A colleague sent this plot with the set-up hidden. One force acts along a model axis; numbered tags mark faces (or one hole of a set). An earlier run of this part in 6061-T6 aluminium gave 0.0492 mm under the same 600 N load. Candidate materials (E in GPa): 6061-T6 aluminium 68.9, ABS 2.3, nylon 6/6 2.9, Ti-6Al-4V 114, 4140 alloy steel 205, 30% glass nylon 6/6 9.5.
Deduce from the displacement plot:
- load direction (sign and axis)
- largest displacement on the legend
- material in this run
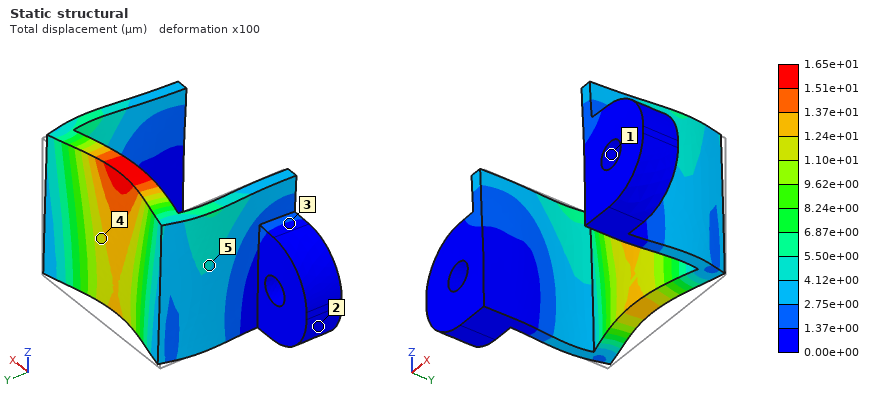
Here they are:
-Y
1.65e+01 µm
4140 alloy steel
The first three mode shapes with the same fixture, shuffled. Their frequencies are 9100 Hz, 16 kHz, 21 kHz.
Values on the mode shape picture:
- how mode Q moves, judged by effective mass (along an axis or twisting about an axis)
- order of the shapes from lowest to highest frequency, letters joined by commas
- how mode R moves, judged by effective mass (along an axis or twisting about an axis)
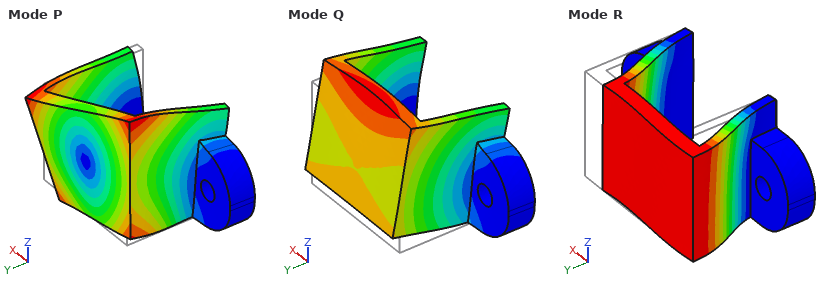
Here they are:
along Z
R, Q, P
along X
